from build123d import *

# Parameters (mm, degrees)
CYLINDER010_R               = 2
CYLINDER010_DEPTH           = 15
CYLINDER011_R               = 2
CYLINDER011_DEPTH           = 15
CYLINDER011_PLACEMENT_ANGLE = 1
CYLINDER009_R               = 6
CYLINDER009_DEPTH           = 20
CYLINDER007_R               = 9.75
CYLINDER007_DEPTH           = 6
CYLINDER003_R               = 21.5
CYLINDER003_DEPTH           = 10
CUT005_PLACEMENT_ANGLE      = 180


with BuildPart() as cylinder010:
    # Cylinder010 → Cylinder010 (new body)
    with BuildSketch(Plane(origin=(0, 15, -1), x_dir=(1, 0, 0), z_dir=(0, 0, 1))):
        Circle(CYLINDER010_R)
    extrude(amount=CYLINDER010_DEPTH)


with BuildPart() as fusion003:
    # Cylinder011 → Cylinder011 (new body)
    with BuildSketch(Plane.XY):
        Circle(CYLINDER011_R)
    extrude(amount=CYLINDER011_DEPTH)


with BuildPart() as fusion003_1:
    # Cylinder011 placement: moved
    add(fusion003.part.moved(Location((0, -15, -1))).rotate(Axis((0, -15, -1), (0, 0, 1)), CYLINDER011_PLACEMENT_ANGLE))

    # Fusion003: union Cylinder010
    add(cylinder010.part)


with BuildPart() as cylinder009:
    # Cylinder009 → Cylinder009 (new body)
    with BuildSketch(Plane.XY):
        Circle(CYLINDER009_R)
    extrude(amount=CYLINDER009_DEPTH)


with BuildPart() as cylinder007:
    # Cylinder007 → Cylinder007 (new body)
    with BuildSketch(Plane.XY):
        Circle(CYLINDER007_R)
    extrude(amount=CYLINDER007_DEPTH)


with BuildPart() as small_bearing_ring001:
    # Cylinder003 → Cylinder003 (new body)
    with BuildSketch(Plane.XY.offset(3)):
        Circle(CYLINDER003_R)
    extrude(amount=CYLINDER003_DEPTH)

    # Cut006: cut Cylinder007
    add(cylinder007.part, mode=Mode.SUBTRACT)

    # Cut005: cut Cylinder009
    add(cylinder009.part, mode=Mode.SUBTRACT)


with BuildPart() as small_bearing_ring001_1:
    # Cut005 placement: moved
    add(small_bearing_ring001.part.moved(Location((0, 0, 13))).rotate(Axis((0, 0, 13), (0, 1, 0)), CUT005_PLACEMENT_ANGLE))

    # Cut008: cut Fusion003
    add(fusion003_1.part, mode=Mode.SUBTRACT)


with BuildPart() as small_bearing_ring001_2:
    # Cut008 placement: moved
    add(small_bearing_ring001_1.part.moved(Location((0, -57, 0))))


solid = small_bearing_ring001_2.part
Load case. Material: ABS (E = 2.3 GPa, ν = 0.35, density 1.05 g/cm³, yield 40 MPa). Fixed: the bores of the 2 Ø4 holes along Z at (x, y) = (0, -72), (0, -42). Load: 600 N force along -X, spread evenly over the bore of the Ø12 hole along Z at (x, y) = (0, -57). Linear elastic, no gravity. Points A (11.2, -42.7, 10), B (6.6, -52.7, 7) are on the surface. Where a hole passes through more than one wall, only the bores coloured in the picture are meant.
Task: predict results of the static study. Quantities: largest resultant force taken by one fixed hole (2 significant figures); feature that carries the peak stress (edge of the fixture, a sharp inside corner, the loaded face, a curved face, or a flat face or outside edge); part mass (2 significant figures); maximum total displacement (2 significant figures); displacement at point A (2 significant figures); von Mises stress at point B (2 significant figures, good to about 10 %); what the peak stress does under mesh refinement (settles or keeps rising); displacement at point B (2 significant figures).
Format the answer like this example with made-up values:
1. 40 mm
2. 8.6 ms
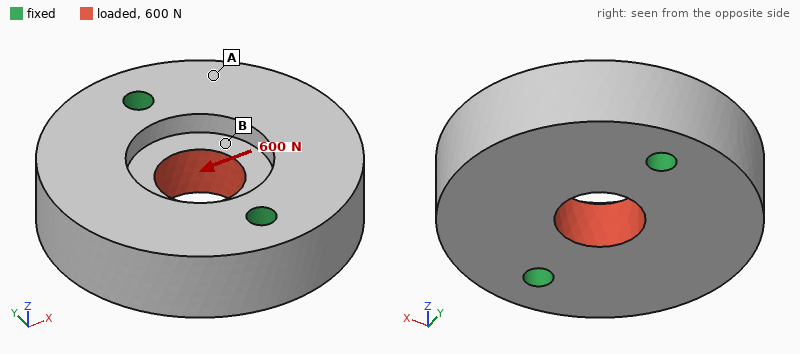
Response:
1. 300 N
2. edge of the fixture
3. 13 g
4. 26 µm
5. 6.9 µm
6. 2.4 MPa
7. keeps rising
8. 15 µm
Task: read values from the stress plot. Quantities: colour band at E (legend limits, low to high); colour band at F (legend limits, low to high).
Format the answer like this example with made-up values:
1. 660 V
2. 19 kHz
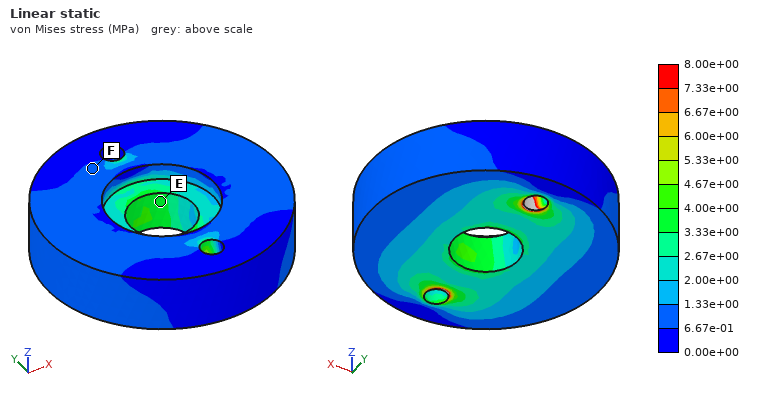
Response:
1. 3.33e+00 to 4.00e+00 MPa
2. 6.67e-01 to 1.33e+00 MPa
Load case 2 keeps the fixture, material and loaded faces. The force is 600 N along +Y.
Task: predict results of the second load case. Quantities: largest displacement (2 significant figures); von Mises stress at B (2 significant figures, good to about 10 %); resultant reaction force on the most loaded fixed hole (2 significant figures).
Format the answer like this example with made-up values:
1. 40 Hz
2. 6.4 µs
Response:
1. 18 µm
2. 2.3 MPa
3. 300 N
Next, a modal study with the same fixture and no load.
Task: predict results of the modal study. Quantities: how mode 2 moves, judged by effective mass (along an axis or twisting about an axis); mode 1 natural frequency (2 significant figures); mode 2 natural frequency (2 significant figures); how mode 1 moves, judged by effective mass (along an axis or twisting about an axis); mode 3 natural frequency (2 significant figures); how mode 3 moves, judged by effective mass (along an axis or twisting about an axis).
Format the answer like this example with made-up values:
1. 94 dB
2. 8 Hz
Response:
1. along Z
2. 4000 Hz
3. 4700 Hz
4. twisting about Y
5. 8600 Hz
6. twisting about Z
